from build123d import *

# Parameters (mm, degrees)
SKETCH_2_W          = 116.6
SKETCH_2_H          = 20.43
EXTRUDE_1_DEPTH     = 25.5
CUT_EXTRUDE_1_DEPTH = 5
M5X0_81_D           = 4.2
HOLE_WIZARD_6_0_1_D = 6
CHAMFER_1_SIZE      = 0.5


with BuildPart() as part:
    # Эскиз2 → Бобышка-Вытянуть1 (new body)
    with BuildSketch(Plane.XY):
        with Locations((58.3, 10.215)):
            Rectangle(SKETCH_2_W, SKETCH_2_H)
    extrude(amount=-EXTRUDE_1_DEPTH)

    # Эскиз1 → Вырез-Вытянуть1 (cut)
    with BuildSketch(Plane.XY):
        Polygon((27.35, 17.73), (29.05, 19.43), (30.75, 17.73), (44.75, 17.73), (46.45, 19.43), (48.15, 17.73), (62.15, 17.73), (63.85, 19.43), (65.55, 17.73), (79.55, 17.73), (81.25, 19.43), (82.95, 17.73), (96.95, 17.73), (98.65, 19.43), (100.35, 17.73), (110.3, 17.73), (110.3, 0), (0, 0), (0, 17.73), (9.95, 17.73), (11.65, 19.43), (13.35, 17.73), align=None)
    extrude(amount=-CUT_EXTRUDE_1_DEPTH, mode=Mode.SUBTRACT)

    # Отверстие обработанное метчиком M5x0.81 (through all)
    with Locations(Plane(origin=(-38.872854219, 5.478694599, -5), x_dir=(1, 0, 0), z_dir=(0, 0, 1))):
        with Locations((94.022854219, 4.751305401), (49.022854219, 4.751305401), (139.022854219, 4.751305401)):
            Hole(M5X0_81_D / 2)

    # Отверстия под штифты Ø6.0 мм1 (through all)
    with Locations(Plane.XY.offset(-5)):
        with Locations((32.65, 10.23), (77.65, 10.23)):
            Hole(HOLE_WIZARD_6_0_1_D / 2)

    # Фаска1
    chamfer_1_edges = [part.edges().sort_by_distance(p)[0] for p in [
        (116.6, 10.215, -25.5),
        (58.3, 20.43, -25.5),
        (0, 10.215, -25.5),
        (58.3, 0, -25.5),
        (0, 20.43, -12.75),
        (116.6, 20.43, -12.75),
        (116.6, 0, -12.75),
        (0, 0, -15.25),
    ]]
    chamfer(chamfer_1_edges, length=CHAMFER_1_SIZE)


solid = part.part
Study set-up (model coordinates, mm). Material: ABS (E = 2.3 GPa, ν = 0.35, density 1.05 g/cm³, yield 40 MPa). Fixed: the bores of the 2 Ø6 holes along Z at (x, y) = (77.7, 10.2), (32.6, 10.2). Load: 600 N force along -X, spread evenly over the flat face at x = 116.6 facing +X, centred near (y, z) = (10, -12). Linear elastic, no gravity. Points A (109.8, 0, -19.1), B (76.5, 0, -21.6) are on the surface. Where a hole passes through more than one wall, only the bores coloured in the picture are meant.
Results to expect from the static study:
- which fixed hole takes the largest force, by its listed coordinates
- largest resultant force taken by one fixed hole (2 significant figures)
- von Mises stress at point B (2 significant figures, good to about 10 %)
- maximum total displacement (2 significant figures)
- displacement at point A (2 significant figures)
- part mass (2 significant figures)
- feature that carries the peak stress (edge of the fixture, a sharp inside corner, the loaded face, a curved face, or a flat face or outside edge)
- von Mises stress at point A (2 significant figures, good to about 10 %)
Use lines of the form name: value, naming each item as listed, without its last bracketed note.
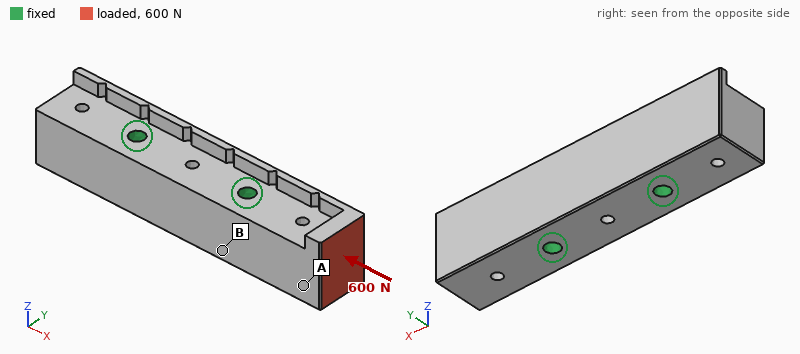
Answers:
which fixed hole takes the largest force, by its listed coordinates: (77.7, 10.2)
largest resultant force taken by one fixed hole: 560 N
von Mises stress at point B: 0.52 MPa
maximum total displacement: 79 µm
displacement at point A: 28 µm
part mass: 51 g
feature that carries the peak stress: a curved face
von Mises stress at point A: 1.1 MPa
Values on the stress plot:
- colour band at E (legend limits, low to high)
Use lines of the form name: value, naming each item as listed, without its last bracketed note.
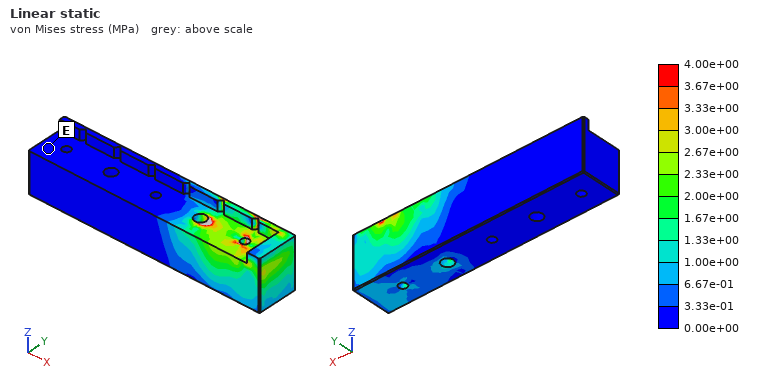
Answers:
colour band at E: 0.00e+00 to 3.33e-01 MPa
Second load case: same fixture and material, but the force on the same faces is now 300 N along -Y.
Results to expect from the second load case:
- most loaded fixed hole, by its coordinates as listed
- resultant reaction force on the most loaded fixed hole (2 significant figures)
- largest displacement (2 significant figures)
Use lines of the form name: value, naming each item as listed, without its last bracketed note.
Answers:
most loaded fixed hole, by its coordinates as listed: (77.7, 10.2)
resultant reaction force on the most loaded fixed hole: 440 N
largest displacement: 0.34 mm
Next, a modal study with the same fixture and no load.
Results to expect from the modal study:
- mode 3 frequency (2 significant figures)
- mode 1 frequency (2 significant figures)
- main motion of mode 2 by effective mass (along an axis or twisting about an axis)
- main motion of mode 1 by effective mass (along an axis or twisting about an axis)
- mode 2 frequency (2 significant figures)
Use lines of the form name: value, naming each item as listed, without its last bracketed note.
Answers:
mode 3 frequency: 2900 Hz
mode 1 frequency: 2100 Hz
main motion of mode 2 by effective mass: along Z
main motion of mode 1 by effective mass: along Y
mode 2 frequency: 2600 Hz
